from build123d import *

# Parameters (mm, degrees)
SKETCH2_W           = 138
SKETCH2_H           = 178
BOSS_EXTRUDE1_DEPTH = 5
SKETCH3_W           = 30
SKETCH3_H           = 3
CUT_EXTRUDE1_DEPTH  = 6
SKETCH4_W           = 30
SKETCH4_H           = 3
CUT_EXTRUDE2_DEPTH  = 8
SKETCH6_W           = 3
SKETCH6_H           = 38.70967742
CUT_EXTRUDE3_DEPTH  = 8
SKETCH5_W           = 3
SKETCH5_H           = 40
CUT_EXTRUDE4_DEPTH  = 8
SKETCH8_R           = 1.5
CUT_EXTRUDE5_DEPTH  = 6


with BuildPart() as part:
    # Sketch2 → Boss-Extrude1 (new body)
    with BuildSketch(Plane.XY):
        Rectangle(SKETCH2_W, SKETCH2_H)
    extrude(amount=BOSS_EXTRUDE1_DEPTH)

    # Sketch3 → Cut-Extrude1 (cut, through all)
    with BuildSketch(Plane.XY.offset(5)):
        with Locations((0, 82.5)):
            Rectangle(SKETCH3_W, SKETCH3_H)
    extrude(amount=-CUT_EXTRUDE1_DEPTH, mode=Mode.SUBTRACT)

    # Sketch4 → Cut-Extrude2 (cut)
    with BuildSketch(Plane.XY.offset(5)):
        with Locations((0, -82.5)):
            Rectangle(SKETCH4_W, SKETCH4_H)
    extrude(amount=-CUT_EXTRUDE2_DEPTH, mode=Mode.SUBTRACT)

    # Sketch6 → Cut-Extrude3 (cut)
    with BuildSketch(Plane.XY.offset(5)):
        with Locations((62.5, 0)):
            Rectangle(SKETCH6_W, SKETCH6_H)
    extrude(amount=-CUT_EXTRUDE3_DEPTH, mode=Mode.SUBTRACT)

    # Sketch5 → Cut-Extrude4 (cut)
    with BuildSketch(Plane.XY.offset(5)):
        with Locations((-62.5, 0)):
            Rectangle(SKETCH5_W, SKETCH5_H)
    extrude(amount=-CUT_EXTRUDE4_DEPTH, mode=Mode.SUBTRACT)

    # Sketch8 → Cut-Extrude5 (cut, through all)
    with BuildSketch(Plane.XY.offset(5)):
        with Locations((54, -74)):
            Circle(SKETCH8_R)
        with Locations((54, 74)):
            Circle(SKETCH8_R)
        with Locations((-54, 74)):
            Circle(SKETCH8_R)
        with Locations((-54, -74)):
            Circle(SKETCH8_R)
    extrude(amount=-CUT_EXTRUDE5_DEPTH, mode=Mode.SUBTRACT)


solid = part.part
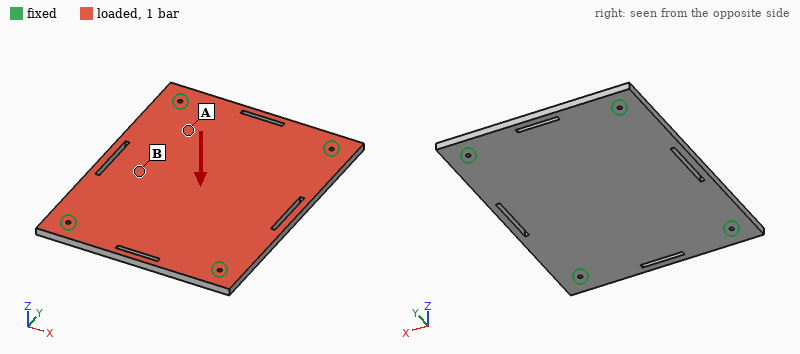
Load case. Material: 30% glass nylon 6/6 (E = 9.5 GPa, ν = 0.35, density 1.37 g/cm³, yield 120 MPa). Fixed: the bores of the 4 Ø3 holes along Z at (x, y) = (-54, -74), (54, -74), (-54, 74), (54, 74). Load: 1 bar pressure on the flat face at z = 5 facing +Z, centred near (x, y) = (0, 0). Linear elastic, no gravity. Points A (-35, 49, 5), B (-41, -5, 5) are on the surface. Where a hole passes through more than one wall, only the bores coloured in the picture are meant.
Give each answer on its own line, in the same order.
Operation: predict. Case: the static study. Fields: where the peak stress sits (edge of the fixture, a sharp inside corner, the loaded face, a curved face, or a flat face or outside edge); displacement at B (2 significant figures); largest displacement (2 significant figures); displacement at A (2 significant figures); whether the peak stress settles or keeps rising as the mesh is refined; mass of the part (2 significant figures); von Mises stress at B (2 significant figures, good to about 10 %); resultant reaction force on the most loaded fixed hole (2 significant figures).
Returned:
edge of the fixture
2.2 mm
2.4 mm
1.1 mm
keeps rising
170 g
27 MPa
600 N
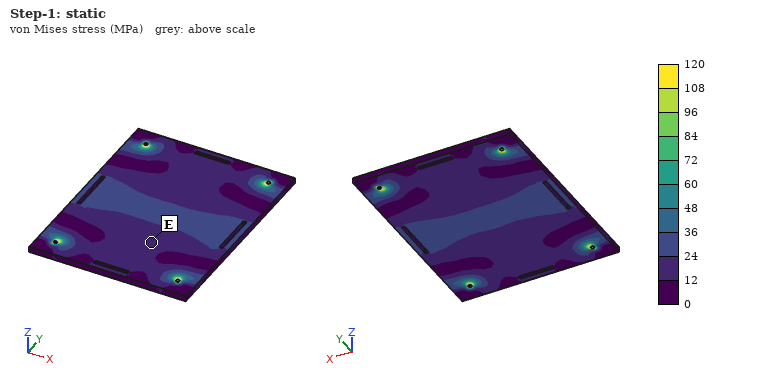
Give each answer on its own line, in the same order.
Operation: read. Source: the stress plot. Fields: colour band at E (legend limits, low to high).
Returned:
12 to 24 MPa
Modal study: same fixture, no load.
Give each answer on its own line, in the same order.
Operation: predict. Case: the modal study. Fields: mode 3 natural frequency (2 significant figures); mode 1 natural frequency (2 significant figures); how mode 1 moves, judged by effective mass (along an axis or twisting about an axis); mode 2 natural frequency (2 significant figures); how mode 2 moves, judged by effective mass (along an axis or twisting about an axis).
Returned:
980 Hz
460 Hz
along Z
700 Hz
twisting about Y
